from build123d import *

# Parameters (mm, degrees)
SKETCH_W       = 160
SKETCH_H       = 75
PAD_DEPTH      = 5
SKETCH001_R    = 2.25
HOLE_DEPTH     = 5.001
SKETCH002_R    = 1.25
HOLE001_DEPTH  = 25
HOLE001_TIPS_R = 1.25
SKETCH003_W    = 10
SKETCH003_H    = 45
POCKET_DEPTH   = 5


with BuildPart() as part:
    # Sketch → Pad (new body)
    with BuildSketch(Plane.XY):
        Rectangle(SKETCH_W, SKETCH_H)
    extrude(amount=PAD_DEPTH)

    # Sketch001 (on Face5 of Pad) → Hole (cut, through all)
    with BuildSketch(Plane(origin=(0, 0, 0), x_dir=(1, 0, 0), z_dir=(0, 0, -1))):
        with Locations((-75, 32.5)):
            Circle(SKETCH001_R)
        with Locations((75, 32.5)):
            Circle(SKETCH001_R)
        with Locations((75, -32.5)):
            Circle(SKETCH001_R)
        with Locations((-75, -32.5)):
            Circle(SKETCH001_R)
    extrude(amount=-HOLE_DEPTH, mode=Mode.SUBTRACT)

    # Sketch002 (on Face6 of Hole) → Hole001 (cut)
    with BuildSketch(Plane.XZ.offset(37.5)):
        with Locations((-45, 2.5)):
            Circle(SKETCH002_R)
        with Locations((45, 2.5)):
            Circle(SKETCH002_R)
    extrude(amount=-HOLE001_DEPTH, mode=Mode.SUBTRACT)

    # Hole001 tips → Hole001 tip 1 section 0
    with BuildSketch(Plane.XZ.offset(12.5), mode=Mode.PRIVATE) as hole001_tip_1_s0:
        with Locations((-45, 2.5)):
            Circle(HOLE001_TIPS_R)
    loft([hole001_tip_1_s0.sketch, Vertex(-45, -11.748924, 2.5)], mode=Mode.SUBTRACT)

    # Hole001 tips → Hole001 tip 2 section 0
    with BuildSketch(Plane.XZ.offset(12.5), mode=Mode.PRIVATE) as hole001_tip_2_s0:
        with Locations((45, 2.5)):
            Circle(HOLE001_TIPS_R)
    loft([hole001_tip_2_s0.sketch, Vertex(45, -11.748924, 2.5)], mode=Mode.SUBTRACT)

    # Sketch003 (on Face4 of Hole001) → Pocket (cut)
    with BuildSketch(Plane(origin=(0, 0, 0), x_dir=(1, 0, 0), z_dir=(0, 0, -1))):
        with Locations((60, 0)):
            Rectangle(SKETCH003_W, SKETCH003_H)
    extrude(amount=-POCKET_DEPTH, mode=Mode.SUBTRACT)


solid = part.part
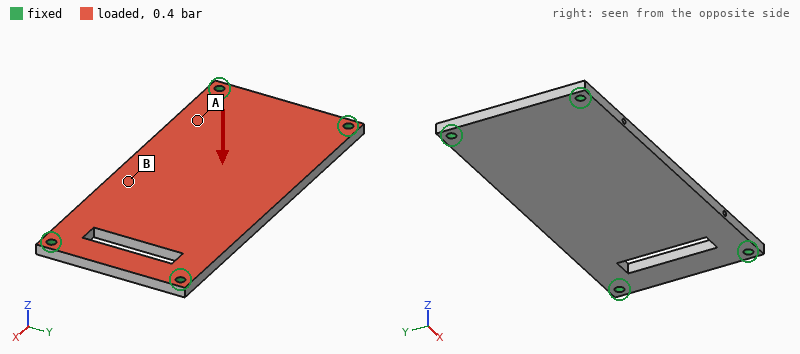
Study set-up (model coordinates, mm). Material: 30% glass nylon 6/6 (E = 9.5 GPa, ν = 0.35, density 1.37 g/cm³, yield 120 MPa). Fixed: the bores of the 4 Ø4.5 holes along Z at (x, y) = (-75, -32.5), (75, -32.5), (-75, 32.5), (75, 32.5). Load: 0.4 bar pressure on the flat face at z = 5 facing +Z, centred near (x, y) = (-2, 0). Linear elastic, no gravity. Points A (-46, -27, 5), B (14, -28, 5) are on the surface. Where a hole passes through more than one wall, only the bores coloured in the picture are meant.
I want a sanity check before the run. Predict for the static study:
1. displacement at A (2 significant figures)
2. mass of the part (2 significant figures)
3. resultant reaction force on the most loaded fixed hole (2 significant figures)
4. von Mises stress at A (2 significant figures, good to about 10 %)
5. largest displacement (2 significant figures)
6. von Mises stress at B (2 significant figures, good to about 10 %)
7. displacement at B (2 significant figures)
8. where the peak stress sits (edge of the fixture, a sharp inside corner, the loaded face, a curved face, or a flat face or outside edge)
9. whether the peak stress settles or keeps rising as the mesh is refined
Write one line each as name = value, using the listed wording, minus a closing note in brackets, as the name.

displacement at A = 0.33 mm
mass of the part = 78 g
resultant reaction force on the most loaded fixed hole = 120 N
von Mises stress at A = 4.3 MPa
largest displacement = 0.79 mm
von Mises stress at B = 11 MPa
displacement at B = 0.72 mm
where the peak stress sits = edge of the fixture
whether the peak stress settles or keeps rising as the mesh is refined = keeps rising
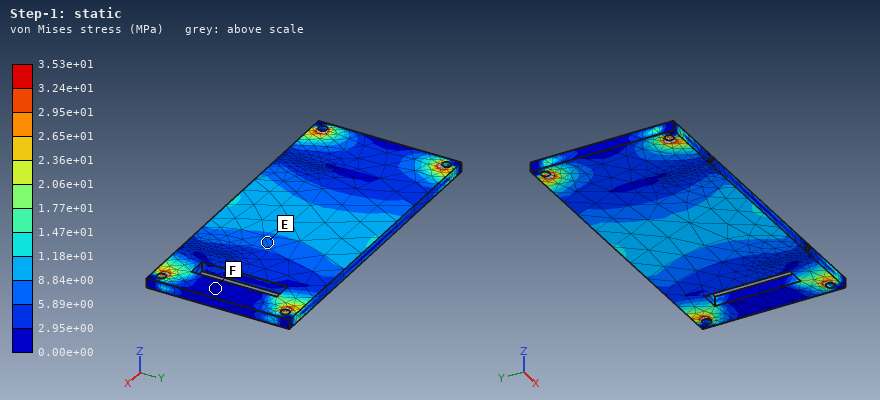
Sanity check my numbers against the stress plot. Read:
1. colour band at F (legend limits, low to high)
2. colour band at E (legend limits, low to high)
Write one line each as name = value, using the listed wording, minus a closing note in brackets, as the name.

colour band at F = 0.00e+00 to 2.95e+00 MPa
colour band at E = 5.89e+00 to 8.84e+00 MPa
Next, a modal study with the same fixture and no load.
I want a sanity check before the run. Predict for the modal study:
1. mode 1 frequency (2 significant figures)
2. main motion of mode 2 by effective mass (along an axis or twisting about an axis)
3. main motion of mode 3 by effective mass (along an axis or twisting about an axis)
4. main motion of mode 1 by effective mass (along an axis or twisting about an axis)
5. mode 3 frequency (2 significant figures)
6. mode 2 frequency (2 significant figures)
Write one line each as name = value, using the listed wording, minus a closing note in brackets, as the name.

mode 1 frequency = 500 Hz
main motion of mode 2 by effective mass = twisting about X
main motion of mode 3 by effective mass = twisting about Y
main motion of mode 1 by effective mass = along Z
mode 3 frequency = 1400 Hz
mode 2 frequency = 940 Hz
